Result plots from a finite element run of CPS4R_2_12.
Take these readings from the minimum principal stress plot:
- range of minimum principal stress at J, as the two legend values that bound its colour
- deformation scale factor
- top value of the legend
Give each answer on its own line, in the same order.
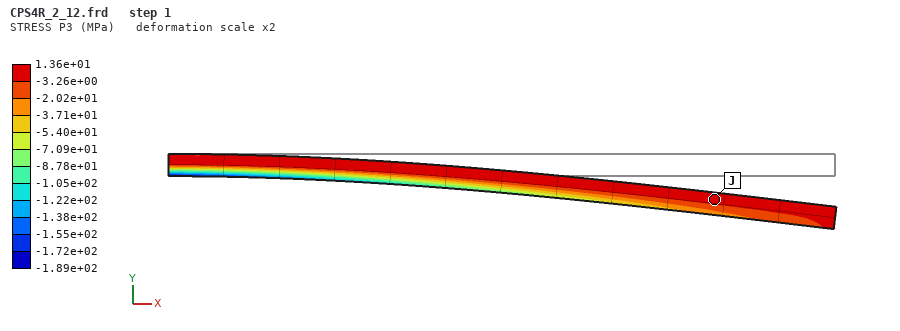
-3.26e+00 to 1.36e+01 MPa
2
1.36e+01 MPa
